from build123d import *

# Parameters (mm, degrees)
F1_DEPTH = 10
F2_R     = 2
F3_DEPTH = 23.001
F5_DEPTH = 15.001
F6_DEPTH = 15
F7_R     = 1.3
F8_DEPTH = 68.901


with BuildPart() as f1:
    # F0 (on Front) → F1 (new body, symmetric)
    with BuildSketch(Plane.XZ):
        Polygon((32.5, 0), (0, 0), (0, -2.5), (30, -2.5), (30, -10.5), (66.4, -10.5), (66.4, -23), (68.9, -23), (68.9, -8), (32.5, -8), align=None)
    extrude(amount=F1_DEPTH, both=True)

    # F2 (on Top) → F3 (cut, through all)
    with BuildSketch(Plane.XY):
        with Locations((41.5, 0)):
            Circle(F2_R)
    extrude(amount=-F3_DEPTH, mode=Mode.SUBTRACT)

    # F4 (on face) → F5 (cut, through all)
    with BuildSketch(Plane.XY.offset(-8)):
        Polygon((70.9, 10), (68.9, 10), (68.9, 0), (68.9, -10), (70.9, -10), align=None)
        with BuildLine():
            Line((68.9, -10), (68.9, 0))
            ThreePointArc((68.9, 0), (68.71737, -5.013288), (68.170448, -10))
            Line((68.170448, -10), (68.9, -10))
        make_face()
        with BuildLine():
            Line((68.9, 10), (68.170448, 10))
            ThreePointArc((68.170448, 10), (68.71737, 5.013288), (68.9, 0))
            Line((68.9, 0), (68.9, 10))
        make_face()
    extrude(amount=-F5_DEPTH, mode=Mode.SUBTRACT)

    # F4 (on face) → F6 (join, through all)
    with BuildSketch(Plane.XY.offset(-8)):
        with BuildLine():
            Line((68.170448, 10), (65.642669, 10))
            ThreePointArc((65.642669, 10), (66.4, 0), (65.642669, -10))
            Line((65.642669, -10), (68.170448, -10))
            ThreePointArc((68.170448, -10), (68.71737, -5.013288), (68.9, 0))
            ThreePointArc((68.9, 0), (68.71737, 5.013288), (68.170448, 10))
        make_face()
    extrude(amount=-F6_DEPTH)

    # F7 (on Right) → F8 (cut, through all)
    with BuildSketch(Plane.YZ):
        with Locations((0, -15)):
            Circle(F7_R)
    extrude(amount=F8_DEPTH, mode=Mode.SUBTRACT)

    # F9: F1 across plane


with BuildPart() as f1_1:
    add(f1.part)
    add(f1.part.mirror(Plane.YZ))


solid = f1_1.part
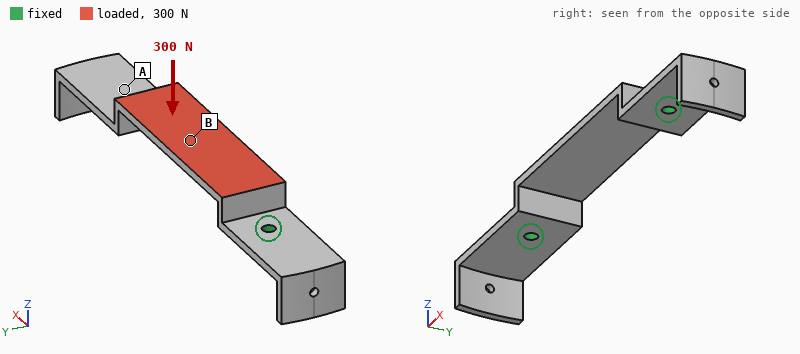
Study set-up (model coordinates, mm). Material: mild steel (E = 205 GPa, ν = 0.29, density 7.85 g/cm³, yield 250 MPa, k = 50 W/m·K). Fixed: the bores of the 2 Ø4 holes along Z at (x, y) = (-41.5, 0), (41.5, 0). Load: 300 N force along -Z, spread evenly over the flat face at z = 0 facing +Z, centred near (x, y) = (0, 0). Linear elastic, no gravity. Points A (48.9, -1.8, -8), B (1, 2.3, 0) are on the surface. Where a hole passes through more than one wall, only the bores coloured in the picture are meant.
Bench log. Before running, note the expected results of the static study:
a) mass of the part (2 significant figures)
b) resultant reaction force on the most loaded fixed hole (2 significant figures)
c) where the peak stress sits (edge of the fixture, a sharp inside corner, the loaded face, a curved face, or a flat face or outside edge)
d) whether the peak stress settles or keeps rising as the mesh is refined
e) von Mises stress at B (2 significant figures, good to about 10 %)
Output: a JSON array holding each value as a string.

["69 g", "310 N", "edge of the fixture", "keeps rising", "42 MPa"]
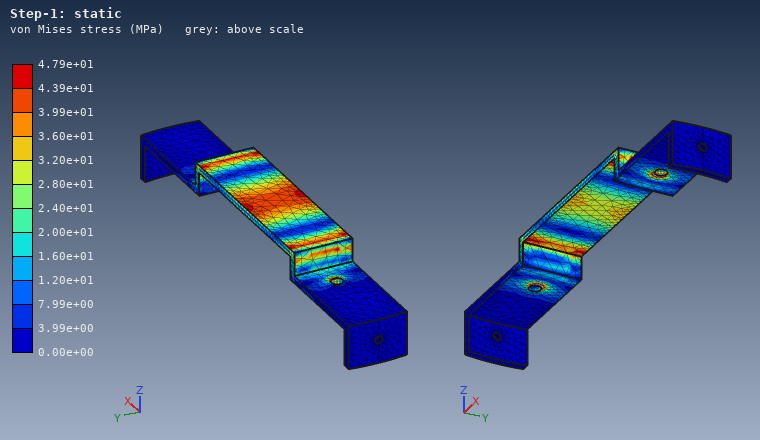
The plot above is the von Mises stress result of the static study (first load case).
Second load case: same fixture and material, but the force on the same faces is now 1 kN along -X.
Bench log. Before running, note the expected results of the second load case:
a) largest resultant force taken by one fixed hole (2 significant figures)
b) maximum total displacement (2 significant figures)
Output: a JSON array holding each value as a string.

["510 N", "42 µm"]
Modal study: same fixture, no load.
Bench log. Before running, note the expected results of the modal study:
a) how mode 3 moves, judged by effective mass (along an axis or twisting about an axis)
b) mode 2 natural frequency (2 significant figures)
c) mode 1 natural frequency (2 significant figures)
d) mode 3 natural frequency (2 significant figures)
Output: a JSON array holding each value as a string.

["along Z", "1700 Hz", "1700 Hz", "3000 Hz"]
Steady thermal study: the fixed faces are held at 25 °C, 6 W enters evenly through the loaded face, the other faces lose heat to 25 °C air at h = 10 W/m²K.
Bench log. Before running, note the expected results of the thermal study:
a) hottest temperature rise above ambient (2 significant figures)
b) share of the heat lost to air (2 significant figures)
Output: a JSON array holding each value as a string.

["35 K", "12 %"]
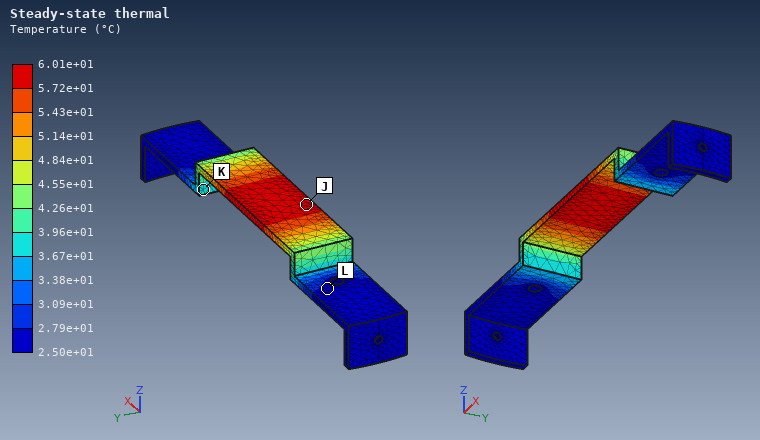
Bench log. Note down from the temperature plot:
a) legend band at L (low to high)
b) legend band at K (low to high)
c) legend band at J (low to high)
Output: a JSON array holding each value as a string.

["2.50e+01 to 2.79e+01 °C", "3.67e+01 to 3.96e+01 °C", "5.72e+01 to 6.01e+01 °C"]
